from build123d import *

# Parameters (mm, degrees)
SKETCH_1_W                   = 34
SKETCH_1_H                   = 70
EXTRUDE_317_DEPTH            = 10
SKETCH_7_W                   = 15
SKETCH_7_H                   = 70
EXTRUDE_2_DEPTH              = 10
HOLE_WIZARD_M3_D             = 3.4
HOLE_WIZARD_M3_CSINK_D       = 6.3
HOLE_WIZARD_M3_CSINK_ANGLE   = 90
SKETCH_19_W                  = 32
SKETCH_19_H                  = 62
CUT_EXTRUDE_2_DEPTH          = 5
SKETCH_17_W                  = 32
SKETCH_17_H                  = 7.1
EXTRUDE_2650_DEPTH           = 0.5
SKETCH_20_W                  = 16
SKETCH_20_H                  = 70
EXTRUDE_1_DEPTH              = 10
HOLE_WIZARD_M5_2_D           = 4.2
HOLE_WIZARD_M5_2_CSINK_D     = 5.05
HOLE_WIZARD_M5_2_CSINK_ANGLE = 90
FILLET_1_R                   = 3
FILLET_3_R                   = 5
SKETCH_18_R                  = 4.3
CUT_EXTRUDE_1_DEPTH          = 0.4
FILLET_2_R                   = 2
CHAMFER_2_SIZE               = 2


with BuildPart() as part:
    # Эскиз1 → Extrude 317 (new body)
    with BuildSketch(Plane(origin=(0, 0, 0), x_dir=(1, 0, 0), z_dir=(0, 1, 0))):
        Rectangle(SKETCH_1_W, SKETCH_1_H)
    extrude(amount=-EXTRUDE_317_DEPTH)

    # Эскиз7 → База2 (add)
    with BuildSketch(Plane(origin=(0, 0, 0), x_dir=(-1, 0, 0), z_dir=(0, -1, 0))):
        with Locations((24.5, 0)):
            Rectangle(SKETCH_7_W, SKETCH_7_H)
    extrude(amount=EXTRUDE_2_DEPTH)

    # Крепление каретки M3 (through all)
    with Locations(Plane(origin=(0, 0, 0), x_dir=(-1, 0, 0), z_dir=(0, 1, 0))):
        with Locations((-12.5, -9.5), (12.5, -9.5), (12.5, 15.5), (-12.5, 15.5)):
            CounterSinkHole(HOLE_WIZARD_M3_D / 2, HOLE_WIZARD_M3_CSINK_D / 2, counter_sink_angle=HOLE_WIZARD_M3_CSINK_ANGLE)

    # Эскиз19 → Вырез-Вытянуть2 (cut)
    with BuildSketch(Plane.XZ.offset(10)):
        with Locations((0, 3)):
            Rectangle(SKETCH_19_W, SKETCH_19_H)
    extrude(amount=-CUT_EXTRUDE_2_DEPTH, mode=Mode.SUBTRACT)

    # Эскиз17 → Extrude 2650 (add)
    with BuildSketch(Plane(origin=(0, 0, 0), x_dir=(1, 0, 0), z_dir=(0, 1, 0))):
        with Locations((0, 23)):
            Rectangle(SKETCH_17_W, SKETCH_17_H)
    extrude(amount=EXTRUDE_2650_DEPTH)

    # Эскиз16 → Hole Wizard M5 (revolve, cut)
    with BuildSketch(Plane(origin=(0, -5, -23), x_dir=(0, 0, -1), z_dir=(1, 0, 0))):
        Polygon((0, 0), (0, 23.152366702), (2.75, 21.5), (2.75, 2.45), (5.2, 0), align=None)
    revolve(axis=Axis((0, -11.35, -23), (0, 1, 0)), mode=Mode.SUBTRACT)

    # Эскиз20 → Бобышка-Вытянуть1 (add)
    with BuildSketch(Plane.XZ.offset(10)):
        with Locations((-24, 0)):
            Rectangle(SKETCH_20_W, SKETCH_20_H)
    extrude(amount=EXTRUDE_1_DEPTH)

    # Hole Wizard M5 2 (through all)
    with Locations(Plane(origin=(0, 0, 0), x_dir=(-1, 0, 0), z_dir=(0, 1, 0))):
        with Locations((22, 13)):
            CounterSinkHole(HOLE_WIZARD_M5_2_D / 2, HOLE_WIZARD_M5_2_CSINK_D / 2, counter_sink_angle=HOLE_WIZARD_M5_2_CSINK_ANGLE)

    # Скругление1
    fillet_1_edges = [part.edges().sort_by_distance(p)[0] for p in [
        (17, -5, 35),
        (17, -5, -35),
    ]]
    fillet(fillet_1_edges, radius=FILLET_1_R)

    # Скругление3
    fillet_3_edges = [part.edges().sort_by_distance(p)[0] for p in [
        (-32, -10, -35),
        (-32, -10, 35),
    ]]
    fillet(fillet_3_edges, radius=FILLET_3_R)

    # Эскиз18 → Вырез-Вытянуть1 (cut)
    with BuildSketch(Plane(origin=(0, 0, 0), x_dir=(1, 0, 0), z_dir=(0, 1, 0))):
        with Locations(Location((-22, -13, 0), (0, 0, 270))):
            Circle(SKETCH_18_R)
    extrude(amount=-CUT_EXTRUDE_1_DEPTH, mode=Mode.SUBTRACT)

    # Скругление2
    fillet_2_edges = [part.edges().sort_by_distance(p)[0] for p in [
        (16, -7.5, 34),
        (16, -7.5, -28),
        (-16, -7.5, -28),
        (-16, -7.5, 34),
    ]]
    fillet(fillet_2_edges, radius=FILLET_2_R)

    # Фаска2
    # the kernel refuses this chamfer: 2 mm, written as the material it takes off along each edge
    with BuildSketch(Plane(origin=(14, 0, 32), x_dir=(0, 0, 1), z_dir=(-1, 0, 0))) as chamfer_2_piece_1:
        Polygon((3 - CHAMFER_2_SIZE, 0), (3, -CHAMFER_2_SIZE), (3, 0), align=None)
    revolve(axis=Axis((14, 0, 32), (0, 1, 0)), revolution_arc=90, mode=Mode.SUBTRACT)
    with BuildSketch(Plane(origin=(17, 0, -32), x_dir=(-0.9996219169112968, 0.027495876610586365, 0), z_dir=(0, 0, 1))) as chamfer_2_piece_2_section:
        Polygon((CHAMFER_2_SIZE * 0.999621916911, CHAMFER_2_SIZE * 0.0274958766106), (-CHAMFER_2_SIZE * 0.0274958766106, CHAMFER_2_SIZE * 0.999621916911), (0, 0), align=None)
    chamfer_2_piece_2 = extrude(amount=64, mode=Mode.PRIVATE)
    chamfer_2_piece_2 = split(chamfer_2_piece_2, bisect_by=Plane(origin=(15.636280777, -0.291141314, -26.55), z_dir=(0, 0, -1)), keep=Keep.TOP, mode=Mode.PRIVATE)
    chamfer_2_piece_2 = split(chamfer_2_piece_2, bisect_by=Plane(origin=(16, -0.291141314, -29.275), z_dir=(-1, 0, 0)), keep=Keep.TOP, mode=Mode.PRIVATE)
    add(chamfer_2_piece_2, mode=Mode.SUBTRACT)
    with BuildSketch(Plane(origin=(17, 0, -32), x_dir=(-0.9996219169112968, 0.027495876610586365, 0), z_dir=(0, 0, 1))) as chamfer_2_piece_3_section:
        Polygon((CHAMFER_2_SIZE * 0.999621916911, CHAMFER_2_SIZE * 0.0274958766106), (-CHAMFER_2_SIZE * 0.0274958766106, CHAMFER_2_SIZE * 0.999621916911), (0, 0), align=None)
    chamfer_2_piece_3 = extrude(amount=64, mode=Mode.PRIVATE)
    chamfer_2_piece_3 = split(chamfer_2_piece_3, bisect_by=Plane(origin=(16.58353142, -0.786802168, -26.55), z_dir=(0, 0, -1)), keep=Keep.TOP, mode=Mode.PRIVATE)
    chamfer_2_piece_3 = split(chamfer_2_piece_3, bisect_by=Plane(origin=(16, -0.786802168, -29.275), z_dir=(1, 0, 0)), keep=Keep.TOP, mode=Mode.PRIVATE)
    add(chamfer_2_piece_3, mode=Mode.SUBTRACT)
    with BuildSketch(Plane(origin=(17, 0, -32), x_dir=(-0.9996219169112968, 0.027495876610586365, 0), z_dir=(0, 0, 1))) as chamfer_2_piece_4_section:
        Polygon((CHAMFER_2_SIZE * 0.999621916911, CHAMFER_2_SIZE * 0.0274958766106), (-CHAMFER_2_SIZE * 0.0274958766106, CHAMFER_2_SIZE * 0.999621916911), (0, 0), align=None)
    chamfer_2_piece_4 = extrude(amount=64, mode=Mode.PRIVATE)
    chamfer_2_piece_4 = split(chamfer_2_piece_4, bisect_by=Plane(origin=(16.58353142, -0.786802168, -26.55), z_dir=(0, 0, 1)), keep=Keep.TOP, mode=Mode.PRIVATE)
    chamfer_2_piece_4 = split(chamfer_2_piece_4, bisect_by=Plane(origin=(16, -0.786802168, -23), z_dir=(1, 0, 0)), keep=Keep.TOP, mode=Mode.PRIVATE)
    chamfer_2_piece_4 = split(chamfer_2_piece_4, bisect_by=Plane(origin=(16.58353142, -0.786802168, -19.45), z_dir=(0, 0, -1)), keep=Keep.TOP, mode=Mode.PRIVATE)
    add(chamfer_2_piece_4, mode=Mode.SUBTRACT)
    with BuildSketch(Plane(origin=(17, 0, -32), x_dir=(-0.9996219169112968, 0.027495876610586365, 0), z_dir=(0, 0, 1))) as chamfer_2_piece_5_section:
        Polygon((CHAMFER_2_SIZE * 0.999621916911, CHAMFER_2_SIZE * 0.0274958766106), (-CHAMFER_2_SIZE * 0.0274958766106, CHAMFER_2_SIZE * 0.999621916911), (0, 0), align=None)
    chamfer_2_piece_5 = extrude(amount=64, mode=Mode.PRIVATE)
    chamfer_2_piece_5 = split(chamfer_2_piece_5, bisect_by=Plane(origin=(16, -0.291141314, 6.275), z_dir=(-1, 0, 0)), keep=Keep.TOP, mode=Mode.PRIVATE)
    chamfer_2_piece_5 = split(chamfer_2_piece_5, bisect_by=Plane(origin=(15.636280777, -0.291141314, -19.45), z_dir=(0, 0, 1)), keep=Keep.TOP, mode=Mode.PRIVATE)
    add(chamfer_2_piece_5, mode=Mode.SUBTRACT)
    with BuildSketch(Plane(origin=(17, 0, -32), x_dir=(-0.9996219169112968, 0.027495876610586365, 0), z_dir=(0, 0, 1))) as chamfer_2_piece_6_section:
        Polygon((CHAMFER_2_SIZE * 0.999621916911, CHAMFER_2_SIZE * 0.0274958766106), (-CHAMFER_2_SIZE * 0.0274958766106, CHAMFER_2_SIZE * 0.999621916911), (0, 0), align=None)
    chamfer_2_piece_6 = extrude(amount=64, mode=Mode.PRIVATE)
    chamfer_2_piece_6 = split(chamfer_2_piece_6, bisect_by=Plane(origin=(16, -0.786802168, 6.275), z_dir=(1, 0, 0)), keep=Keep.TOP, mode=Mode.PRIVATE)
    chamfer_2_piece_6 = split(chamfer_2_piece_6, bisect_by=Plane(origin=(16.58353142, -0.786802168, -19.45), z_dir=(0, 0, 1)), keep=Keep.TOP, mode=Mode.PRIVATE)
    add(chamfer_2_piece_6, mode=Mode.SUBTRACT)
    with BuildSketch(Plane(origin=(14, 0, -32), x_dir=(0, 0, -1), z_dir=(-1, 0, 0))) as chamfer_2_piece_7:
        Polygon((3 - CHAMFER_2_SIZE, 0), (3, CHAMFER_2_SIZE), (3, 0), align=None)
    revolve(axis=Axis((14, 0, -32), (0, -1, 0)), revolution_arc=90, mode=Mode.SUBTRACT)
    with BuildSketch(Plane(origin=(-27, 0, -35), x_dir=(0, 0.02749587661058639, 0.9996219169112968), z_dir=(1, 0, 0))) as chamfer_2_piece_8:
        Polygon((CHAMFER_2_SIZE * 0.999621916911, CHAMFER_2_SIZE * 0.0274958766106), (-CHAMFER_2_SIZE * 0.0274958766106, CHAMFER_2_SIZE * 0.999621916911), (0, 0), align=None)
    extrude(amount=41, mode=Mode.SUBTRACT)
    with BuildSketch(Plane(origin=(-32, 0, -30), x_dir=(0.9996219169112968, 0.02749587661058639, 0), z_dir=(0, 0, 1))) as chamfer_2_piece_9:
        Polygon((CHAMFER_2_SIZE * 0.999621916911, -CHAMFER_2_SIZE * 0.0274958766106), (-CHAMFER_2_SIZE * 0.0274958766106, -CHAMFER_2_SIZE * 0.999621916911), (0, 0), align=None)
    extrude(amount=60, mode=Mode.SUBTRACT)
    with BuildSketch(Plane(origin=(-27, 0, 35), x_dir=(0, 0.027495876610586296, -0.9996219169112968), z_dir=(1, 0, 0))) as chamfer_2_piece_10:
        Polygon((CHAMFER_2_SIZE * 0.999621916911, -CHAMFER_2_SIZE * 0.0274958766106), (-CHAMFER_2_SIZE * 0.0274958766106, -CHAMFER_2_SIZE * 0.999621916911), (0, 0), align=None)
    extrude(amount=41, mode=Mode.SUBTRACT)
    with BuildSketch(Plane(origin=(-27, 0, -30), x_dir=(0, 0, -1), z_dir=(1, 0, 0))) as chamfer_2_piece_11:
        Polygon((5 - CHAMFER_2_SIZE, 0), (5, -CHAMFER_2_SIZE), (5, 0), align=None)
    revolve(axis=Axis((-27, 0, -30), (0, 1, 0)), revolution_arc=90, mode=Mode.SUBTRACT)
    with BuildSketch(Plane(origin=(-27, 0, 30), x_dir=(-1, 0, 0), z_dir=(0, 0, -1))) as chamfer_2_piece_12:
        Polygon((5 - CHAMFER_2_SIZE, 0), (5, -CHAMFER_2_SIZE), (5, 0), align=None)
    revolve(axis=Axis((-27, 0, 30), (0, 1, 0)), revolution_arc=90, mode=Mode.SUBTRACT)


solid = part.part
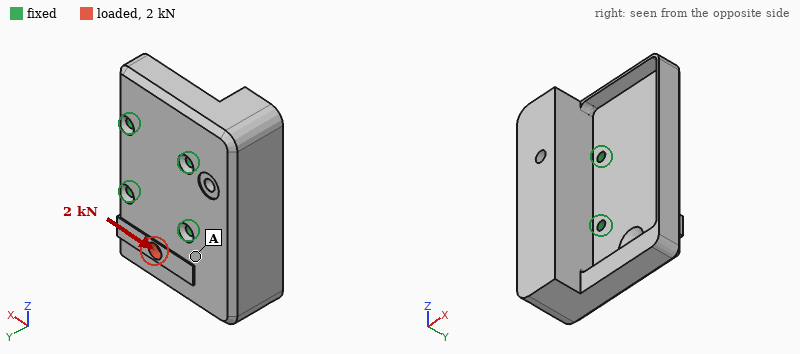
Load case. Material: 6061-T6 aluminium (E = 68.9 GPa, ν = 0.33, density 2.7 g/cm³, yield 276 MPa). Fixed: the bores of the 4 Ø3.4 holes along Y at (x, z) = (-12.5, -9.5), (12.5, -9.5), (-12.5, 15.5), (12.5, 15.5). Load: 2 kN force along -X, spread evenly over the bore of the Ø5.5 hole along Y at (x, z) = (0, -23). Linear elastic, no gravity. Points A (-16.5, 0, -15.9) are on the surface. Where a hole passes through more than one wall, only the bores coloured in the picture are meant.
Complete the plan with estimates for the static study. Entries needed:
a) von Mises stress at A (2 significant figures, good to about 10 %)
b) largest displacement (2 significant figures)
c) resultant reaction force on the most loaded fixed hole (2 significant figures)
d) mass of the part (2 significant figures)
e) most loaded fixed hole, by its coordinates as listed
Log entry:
9.5 MPa
12 µm
1.4 kN
93 g
(-12.5, -9.5)
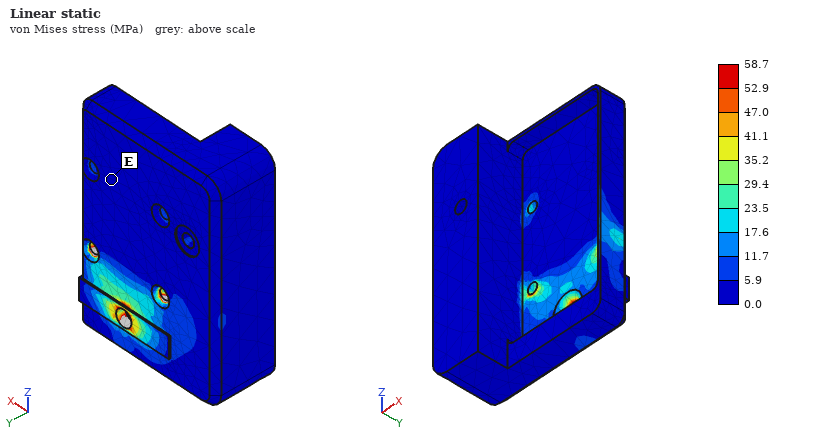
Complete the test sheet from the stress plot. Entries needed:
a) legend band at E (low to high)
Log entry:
0.0 to 5.9 MPa
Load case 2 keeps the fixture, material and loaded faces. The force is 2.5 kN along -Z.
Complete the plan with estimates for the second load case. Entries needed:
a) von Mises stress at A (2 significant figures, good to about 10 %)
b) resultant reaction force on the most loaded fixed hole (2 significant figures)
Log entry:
9.2 MPa
1.1 kN
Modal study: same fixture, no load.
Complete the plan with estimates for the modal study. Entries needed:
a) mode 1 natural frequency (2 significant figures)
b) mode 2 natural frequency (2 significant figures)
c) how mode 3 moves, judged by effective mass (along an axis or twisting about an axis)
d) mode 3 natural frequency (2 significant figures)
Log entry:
3600 Hz
5400 Hz
along Y
8300 Hz
